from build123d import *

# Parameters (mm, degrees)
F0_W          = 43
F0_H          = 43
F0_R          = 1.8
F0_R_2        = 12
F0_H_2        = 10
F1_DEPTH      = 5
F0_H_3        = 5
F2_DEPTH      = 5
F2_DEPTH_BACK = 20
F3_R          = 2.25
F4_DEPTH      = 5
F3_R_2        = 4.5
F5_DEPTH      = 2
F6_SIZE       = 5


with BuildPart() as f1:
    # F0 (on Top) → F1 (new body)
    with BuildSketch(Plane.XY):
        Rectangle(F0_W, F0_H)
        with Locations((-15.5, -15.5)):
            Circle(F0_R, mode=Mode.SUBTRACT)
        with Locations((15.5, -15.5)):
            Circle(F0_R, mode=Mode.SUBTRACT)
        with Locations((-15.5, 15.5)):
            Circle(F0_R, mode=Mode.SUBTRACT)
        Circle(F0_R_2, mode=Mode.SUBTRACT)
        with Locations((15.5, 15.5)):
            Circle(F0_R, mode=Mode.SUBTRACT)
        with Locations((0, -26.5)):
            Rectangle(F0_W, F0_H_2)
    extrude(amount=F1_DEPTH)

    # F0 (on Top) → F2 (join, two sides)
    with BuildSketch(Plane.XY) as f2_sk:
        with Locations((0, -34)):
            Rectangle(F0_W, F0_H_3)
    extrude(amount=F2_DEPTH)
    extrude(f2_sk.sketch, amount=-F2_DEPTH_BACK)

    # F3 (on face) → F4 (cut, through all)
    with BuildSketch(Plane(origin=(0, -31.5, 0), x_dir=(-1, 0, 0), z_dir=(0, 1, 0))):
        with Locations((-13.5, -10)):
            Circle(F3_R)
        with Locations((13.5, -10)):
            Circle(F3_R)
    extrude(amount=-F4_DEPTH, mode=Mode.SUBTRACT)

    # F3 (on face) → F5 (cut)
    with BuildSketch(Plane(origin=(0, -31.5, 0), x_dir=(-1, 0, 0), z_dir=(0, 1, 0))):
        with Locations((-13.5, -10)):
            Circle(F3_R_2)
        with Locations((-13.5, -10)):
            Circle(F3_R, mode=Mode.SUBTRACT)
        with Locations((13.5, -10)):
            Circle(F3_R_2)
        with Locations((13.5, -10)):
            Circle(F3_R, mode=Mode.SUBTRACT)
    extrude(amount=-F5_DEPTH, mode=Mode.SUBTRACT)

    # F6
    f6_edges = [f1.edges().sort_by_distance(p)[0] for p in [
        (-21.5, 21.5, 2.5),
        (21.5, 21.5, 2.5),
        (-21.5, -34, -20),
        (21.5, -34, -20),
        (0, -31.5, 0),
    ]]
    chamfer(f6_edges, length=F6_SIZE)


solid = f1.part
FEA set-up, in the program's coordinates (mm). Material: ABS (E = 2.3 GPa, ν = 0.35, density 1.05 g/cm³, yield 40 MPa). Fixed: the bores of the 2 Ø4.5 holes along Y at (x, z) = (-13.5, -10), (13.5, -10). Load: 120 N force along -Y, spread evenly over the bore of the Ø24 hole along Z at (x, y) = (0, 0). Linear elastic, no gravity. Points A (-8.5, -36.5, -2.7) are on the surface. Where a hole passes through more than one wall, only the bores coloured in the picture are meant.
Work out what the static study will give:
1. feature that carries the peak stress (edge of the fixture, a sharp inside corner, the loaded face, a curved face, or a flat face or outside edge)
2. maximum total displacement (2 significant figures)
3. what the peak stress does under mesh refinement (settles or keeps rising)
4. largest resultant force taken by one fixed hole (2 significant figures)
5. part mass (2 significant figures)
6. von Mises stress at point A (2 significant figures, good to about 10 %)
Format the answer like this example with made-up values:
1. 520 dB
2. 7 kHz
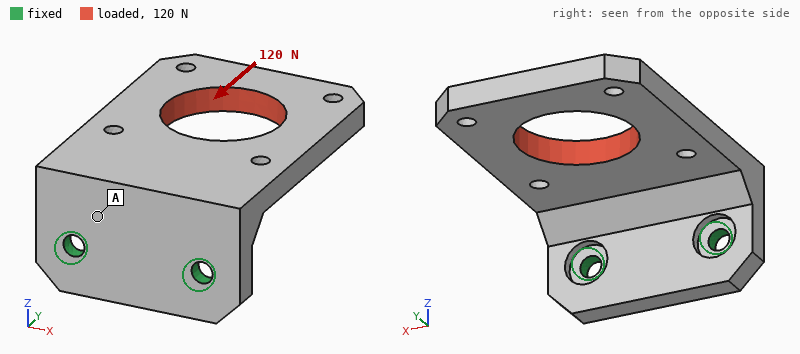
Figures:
1. edge of the fixture
2. 0.90 mm
3. keeps rising
4. 60 N
5. 15 g
6. 2.8 MPa
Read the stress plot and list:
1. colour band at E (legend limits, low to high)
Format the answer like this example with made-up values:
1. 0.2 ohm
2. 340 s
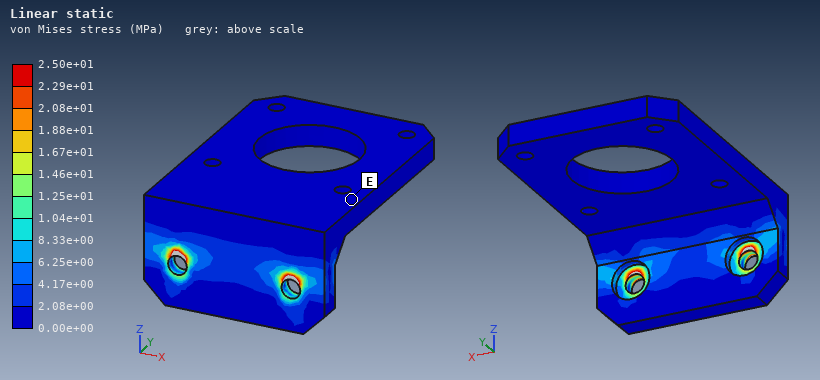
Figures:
1. 0.00e+00 to 2.08e+00 MPa
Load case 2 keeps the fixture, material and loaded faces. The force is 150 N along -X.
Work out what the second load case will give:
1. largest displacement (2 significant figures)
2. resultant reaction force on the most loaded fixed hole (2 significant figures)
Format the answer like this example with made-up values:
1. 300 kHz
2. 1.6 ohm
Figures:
1. 0.72 mm
2. 210 N
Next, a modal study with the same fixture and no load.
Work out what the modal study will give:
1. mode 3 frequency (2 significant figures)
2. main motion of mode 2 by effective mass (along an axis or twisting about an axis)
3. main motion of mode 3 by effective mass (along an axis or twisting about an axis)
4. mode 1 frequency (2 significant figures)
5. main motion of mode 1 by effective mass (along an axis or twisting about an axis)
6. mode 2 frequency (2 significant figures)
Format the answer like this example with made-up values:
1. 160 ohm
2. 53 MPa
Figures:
1. 1200 Hz
2. along X
3. along X
4. 320 Hz
5. along Z
6. 880 Hz
